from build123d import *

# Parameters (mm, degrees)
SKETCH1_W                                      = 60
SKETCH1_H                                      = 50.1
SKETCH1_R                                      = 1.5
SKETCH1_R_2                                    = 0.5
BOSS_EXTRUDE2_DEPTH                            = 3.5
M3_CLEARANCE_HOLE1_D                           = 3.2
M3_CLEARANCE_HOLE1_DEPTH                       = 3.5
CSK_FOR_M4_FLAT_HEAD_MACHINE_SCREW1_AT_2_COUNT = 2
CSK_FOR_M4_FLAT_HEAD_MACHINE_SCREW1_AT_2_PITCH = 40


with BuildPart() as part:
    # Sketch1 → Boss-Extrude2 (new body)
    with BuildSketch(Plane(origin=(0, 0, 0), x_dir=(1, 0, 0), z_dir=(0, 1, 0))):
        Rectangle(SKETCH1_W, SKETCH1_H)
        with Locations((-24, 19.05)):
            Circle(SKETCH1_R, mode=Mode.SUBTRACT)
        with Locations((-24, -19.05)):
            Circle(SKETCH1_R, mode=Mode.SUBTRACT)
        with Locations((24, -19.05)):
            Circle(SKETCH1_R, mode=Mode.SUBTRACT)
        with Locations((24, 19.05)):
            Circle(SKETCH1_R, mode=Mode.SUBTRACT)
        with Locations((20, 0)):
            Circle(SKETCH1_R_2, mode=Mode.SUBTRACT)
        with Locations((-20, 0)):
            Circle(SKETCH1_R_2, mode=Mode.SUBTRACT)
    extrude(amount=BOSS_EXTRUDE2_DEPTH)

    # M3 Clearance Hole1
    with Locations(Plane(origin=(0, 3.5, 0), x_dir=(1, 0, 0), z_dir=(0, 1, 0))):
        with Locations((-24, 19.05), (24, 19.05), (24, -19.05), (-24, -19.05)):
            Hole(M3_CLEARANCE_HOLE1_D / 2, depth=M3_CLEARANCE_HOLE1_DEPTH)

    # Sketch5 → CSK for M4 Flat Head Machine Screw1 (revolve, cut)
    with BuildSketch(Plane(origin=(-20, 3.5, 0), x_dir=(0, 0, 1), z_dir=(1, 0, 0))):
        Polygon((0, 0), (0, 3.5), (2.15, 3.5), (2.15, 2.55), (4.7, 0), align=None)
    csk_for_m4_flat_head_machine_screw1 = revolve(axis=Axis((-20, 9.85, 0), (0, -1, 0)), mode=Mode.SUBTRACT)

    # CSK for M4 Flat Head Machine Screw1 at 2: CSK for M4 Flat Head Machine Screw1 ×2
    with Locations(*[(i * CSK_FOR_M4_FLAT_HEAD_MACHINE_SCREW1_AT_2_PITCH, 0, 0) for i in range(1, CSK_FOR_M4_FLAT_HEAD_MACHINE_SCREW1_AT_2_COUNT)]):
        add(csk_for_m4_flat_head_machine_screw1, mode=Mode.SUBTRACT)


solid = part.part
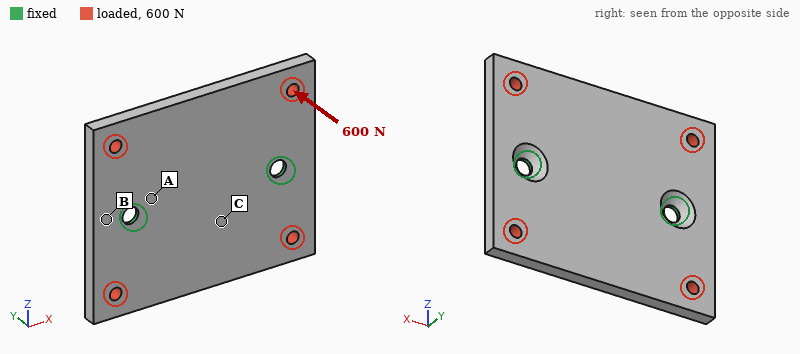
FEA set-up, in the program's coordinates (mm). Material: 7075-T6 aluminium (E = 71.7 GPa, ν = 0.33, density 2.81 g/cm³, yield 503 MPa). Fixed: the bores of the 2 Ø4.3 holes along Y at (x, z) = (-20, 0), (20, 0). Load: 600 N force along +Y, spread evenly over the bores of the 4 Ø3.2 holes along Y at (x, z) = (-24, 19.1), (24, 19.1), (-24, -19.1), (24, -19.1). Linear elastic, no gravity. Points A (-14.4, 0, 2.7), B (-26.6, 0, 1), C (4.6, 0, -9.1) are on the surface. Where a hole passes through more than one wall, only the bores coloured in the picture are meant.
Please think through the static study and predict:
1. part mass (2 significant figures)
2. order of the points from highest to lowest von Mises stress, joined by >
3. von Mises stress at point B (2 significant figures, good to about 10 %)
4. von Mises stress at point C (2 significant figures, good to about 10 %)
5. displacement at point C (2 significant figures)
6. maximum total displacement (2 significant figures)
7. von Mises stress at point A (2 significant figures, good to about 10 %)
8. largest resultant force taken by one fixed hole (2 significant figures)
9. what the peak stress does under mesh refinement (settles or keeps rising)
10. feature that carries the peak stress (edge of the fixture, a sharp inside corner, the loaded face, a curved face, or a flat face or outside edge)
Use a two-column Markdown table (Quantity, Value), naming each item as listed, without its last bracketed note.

| Quantity | Value |
|---|---|
| part mass | 29 g |
| order of the points from highest to lowest von Mises stress, joined by > | B > A > C |
| von Mises stress at point B | 51 MPa |
| von Mises stress at point C | 20 MPa |
| displacement at point C | 14 µm |
| maximum total displacement | 90 µm |
| von Mises stress at point A | 37 MPa |
| largest resultant force taken by one fixed hole | 300 N |
| what the peak stress does under mesh refinement | keeps rising |
| feature that carries the peak stress | edge of the fixture |
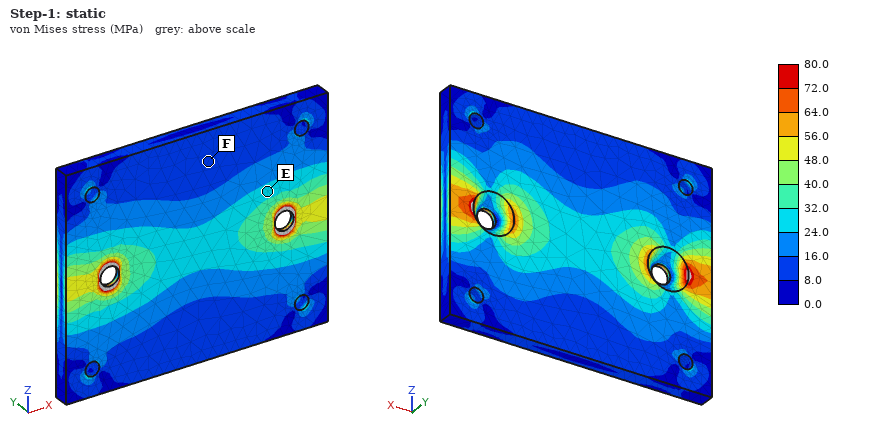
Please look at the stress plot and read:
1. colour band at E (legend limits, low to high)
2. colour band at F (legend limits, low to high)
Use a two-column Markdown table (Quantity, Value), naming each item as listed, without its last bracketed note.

| Quantity | Value |
|---|---|
| colour band at E | 24.0 to 32.0 MPa |
| colour band at F | 8.0 to 16.0 MPa |
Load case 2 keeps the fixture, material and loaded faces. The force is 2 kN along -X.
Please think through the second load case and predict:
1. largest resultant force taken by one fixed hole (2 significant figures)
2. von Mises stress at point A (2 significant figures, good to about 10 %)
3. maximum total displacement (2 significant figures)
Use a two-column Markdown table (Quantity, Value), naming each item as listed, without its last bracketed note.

| Quantity | Value |
|---|---|
| largest resultant force taken by one fixed hole | 1.0 kN |
| von Mises stress at point A | 29 MPa |
| maximum total displacement | 10 µm |
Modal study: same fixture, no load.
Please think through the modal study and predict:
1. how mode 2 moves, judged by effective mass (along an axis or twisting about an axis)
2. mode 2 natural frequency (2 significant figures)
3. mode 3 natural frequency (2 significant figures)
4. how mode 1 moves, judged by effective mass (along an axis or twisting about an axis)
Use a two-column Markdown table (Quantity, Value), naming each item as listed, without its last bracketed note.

| Quantity | Value |
|---|---|
| how mode 2 moves, judged by effective mass | along Y |
| mode 2 natural frequency | 4000 Hz |
| mode 3 natural frequency | 4400 Hz |
| how mode 1 moves, judged by effective mass | twisting about X |
